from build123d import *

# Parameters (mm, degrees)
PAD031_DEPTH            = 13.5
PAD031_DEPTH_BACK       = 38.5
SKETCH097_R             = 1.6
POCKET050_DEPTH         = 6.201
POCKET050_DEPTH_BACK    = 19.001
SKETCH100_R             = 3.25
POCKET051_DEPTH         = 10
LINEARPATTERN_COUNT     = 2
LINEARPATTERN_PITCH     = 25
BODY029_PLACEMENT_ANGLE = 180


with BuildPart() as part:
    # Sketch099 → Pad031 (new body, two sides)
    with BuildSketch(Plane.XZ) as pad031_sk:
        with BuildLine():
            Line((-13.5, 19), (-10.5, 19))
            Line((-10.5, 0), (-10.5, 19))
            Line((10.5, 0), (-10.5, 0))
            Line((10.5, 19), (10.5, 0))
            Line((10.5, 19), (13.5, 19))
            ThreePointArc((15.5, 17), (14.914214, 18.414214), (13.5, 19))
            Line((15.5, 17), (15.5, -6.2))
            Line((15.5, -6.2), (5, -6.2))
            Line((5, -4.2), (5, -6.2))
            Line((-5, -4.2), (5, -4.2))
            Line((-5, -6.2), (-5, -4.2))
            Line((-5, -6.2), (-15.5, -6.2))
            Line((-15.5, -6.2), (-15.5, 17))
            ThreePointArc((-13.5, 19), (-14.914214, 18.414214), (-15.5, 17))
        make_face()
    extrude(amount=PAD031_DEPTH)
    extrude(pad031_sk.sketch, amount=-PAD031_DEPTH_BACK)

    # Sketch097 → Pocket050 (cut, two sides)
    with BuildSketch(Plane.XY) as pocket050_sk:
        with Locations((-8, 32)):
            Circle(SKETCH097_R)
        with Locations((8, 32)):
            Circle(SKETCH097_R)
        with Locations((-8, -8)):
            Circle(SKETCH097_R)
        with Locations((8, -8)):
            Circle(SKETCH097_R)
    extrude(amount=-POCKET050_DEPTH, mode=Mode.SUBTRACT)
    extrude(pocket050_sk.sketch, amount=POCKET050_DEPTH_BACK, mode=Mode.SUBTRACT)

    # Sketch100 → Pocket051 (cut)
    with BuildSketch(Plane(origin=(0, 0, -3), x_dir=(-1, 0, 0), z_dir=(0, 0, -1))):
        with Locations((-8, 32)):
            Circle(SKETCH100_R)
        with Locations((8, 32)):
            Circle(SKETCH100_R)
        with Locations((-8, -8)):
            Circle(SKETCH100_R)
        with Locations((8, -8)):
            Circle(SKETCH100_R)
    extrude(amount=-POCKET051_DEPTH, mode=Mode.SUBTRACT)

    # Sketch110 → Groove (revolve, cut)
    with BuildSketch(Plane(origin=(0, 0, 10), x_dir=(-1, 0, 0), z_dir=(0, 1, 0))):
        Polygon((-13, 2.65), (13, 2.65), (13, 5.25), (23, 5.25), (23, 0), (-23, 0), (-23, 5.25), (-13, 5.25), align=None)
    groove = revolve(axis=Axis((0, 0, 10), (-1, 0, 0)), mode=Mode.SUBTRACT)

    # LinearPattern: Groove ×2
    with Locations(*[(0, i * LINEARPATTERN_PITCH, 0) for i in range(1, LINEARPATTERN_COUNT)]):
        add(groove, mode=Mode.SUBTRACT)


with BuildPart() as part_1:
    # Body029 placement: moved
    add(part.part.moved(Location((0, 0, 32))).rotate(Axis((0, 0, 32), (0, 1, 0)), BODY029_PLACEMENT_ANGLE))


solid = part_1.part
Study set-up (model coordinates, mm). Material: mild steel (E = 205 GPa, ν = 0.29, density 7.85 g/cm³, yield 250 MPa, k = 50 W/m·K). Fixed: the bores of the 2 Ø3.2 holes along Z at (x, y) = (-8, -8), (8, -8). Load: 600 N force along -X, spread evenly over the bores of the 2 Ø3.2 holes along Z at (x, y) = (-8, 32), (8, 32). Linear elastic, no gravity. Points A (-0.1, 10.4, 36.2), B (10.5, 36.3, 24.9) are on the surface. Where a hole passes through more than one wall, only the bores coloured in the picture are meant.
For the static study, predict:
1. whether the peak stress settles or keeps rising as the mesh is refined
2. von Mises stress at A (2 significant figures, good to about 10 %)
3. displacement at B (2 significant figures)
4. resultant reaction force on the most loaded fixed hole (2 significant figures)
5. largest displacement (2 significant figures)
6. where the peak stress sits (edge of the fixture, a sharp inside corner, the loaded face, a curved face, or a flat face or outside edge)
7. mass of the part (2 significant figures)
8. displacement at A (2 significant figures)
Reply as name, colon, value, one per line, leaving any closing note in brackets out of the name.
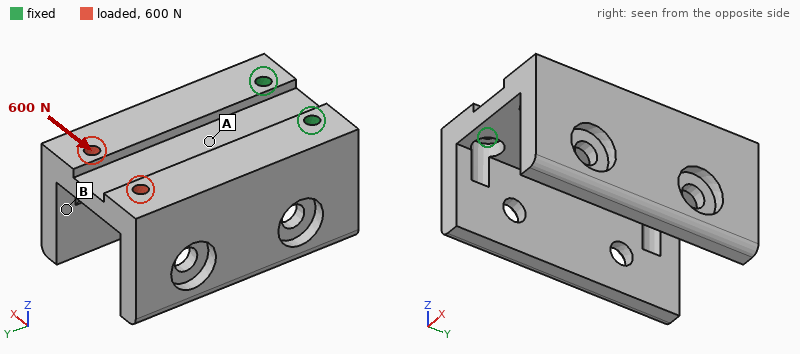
whether the peak stress settles or keeps rising as the mesh is refined: keeps rising
von Mises stress at A: 19 MPa
displacement at B: 11 µm
resultant reaction force on the most loaded fixed hole: 1.3 kN
largest displacement: 18 µm
where the peak stress sits: edge of the fixture
mass of the part: 130 g
displacement at A: 5.3 µm
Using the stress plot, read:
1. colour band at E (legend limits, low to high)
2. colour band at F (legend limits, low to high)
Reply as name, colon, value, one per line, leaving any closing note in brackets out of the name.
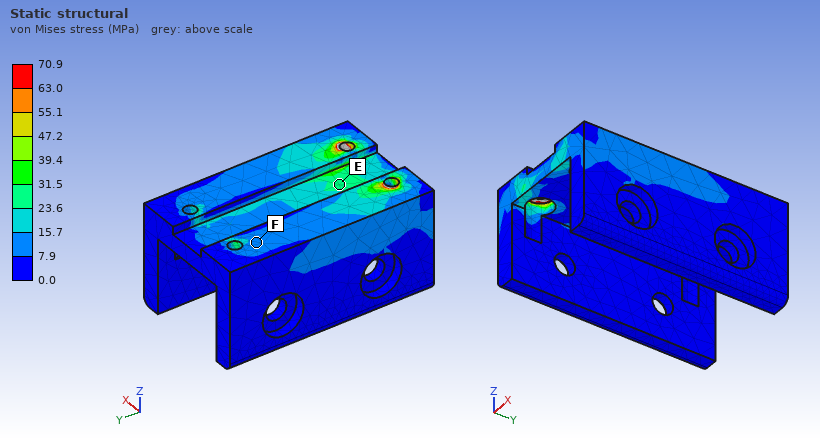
colour band at E: 23.6 to 31.5 MPa
colour band at F: 7.9 to 15.7 MPa
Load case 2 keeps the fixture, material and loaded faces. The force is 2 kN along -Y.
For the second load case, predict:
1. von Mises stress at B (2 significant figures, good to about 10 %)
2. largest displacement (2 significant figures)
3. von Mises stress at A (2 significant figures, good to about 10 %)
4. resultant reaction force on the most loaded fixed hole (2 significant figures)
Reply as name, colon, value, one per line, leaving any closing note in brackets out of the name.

von Mises stress at B: 5.3 MPa
largest displacement: 8.4 µm
von Mises stress at A: 12 MPa
resultant reaction force on the most loaded fixed hole: 1.0 kN
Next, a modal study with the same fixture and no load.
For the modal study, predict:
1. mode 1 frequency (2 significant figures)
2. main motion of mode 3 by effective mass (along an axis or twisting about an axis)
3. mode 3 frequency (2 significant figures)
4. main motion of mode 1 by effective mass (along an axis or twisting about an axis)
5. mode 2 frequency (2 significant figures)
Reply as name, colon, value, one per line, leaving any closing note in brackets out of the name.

mode 1 frequency: 1500 Hz
main motion of mode 3 by effective mass: along X
mode 3 frequency: 4700 Hz
main motion of mode 1 by effective mass: along Z
mode 2 frequency: 3000 Hz
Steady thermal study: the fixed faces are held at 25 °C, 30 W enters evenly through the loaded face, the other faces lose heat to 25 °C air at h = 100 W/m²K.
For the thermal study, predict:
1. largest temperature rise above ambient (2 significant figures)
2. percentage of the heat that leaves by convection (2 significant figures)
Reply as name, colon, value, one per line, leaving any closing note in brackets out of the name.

largest temperature rise above ambient: 73 K
percentage of the heat that leaves by convection: 70 %
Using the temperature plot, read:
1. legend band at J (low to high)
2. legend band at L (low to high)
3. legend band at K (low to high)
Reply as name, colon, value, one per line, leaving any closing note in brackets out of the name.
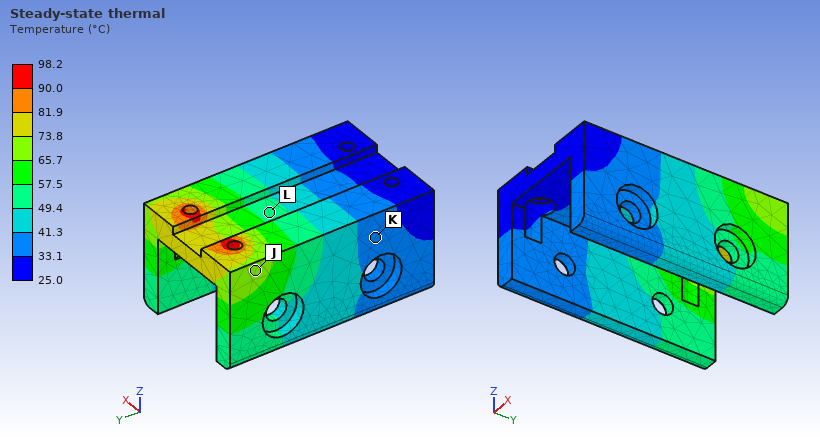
legend band at J: 65.7 to 73.8 °C
legend band at L: 49.4 to 57.5 °C
legend band at K: 33.1 to 41.3 °C
